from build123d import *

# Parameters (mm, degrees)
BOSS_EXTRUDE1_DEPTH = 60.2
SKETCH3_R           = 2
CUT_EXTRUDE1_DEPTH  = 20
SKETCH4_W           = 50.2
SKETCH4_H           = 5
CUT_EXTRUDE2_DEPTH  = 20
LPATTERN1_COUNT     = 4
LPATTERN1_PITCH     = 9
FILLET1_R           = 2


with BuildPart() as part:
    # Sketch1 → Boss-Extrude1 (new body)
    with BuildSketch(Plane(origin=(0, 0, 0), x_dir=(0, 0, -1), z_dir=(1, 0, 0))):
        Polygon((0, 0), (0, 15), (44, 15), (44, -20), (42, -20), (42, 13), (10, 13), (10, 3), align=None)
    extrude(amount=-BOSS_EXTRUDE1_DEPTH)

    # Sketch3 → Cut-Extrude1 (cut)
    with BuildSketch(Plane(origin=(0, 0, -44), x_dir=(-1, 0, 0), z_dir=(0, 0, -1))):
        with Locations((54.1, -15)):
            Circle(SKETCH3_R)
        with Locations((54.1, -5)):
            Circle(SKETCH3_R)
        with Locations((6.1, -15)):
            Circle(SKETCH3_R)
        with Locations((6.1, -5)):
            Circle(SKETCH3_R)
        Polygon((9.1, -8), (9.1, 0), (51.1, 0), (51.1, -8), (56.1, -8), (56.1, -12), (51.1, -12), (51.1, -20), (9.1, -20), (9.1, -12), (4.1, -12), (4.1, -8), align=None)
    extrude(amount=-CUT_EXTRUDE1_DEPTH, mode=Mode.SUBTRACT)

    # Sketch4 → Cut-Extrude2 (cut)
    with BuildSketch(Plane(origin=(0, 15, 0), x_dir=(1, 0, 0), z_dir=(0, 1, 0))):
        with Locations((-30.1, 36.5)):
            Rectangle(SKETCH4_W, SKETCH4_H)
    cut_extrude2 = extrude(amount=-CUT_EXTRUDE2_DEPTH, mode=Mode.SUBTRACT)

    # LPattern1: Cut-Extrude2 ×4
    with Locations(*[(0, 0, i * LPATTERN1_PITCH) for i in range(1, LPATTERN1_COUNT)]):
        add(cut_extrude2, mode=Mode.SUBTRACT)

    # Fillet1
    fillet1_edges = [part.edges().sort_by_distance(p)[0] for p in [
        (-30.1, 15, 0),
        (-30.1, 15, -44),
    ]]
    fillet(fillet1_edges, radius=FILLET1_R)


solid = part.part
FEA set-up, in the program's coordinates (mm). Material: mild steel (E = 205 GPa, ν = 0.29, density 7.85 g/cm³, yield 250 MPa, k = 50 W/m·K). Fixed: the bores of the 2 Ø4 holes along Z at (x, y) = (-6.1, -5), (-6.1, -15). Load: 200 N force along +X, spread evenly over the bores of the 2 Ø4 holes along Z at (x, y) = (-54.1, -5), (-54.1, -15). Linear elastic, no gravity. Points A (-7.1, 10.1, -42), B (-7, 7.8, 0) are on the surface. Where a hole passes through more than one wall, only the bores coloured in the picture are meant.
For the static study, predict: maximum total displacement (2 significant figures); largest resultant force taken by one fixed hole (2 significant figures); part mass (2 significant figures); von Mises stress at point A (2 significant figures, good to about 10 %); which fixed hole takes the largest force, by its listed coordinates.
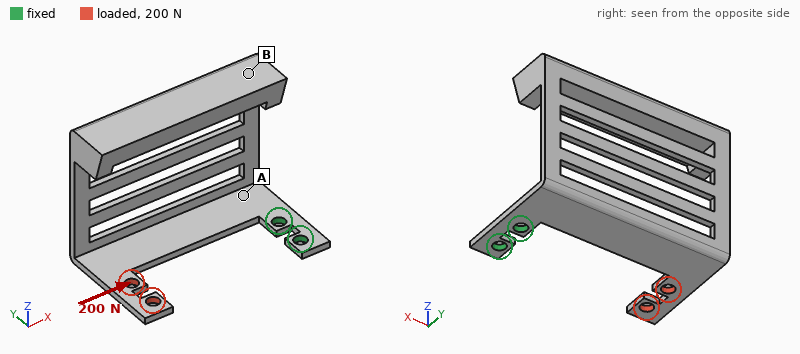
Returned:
0.14 mm
180 N
84 g
24 MPa
(-6.1, -5)
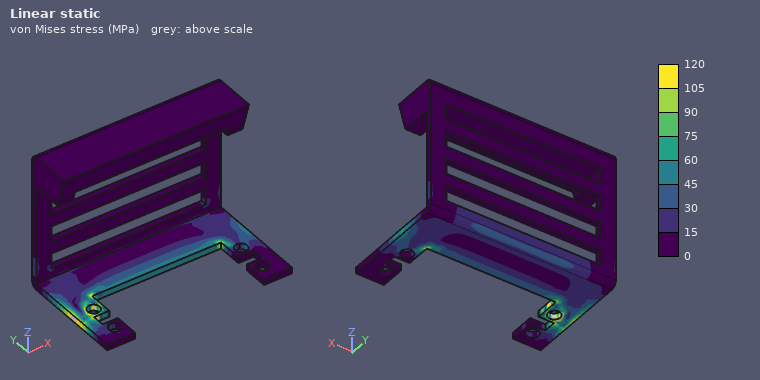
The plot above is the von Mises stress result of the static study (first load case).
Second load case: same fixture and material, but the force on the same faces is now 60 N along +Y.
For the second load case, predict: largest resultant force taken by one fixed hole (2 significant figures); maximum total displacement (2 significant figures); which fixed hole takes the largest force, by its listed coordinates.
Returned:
200 N
93 µm
(-6.1, -5)
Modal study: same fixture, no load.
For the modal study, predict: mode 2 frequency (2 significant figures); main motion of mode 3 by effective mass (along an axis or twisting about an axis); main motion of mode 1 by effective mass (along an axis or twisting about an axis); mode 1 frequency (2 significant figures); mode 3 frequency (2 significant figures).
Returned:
150 Hz
along Z
along Y
120 Hz
590 Hz
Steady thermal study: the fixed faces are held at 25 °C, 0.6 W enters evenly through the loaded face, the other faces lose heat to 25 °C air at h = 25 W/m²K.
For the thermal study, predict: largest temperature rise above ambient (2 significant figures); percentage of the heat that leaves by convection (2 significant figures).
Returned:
19 K
80 %
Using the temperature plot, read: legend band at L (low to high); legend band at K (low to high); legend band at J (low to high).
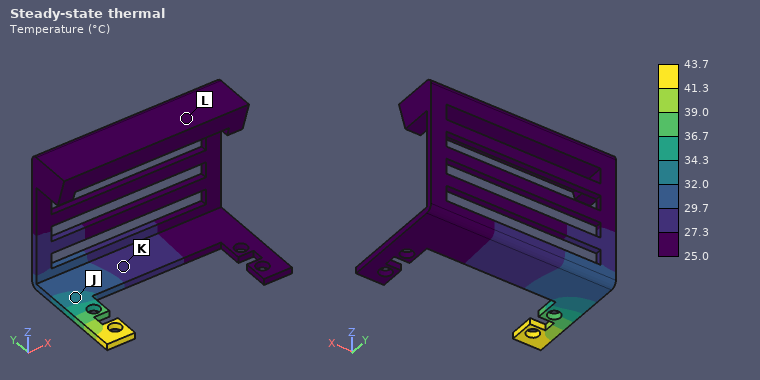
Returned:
25.0 to 27.3 °C
27.3 to 29.7 °C
32.0 to 34.3 °C
